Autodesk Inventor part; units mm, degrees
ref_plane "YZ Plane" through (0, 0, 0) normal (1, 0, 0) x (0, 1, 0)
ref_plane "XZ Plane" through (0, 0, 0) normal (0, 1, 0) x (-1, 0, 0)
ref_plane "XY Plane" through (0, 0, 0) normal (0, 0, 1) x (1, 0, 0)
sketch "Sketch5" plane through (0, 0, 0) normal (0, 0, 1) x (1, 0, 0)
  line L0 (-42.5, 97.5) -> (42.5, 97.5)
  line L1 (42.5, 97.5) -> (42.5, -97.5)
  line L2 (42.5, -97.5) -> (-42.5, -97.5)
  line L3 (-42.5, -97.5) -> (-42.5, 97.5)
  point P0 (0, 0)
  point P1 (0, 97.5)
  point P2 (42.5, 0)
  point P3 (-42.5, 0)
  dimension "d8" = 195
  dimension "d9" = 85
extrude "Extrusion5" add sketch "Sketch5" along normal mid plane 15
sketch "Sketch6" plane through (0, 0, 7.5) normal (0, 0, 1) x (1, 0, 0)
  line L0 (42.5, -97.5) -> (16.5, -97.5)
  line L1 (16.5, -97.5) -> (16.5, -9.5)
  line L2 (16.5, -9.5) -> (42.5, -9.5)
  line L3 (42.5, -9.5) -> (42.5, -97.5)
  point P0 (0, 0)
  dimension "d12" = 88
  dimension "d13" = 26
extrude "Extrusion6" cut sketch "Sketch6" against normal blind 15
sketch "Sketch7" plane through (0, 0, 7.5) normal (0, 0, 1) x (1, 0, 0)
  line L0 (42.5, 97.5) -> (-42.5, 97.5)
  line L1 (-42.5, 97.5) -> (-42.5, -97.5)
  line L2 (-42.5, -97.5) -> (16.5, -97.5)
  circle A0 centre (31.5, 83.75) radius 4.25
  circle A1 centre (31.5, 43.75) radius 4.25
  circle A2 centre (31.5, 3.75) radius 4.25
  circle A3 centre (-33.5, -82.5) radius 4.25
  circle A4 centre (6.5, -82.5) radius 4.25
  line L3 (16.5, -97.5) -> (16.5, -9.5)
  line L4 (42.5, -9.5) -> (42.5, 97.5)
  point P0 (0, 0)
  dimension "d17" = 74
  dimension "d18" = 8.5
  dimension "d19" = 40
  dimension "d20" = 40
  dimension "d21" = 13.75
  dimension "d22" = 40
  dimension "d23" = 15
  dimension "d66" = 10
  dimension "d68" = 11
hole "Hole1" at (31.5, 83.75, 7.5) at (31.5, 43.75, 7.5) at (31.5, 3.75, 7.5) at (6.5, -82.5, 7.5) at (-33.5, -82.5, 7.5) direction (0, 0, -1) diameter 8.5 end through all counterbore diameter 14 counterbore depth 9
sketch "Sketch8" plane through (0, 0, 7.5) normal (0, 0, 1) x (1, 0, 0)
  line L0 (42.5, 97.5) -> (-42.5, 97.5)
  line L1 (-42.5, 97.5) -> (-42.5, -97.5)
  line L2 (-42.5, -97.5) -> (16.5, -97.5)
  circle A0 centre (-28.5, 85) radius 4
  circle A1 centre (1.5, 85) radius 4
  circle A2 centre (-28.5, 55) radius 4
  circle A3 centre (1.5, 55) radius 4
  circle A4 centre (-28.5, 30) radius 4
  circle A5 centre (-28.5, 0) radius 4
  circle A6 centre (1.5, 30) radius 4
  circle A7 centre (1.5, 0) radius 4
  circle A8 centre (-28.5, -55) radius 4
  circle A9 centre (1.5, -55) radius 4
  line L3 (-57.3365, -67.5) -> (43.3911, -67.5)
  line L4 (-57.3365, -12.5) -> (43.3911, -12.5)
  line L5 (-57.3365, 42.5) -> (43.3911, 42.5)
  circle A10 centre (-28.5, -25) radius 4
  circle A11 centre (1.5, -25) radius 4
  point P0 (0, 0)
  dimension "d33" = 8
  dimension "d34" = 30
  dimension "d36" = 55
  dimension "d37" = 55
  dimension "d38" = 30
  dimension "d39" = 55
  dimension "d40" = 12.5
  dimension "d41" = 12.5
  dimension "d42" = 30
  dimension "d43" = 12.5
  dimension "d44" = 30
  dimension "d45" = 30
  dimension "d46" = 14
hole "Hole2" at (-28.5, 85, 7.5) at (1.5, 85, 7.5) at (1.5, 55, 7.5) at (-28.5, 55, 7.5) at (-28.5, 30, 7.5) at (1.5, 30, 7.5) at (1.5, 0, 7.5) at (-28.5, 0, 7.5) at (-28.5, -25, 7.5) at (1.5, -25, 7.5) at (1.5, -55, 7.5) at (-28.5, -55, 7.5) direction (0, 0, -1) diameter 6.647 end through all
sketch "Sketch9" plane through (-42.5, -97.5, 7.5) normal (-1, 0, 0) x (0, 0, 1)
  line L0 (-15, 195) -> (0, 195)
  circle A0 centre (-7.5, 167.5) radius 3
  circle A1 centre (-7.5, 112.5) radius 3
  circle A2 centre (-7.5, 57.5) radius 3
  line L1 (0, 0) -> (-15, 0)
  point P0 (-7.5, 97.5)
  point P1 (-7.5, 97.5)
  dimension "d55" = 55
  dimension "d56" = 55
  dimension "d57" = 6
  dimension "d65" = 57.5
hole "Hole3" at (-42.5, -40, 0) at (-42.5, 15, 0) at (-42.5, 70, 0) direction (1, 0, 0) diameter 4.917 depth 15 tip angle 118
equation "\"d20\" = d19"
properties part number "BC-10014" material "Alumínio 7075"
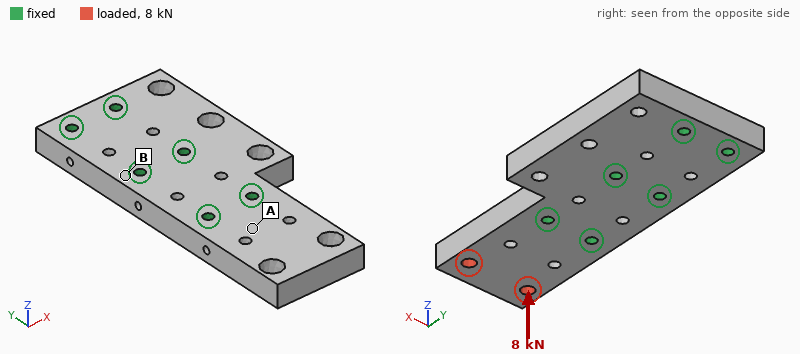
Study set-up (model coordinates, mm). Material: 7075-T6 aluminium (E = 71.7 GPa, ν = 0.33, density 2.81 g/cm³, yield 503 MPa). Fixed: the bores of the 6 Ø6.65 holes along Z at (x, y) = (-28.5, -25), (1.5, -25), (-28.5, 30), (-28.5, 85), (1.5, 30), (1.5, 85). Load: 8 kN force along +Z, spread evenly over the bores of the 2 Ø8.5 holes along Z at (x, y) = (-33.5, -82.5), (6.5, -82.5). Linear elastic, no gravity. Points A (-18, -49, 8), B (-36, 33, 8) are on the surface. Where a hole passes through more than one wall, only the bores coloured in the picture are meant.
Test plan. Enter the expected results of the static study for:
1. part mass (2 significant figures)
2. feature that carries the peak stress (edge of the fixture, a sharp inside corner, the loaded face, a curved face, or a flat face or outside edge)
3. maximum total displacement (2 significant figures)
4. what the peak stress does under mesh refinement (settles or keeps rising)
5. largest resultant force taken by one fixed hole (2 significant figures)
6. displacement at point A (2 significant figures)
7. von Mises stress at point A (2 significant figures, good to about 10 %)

560 g
edge of the fixture
0.67 mm
keeps rising
5.1 kN
0.13 mm
120 MPa
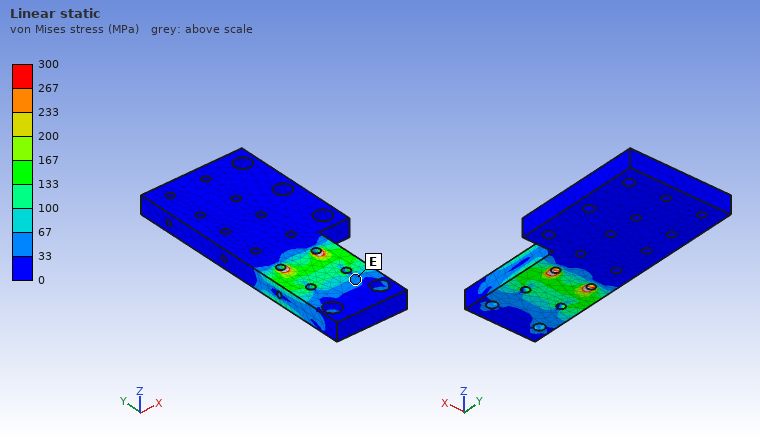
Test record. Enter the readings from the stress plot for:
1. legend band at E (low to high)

33 to 67 MPa
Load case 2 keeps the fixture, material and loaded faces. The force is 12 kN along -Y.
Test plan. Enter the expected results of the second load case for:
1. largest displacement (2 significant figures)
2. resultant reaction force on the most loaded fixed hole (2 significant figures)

0.13 mm
5.6 kN
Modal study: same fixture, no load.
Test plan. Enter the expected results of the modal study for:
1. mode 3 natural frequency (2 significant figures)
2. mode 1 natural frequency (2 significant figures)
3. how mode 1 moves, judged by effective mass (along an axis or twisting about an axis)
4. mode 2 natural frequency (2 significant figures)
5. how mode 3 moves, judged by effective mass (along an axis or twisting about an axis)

6000 Hz
2300 Hz
along Z
5700 Hz
along X
